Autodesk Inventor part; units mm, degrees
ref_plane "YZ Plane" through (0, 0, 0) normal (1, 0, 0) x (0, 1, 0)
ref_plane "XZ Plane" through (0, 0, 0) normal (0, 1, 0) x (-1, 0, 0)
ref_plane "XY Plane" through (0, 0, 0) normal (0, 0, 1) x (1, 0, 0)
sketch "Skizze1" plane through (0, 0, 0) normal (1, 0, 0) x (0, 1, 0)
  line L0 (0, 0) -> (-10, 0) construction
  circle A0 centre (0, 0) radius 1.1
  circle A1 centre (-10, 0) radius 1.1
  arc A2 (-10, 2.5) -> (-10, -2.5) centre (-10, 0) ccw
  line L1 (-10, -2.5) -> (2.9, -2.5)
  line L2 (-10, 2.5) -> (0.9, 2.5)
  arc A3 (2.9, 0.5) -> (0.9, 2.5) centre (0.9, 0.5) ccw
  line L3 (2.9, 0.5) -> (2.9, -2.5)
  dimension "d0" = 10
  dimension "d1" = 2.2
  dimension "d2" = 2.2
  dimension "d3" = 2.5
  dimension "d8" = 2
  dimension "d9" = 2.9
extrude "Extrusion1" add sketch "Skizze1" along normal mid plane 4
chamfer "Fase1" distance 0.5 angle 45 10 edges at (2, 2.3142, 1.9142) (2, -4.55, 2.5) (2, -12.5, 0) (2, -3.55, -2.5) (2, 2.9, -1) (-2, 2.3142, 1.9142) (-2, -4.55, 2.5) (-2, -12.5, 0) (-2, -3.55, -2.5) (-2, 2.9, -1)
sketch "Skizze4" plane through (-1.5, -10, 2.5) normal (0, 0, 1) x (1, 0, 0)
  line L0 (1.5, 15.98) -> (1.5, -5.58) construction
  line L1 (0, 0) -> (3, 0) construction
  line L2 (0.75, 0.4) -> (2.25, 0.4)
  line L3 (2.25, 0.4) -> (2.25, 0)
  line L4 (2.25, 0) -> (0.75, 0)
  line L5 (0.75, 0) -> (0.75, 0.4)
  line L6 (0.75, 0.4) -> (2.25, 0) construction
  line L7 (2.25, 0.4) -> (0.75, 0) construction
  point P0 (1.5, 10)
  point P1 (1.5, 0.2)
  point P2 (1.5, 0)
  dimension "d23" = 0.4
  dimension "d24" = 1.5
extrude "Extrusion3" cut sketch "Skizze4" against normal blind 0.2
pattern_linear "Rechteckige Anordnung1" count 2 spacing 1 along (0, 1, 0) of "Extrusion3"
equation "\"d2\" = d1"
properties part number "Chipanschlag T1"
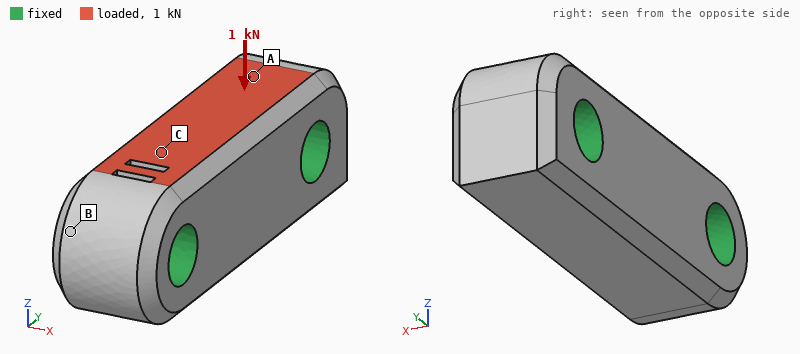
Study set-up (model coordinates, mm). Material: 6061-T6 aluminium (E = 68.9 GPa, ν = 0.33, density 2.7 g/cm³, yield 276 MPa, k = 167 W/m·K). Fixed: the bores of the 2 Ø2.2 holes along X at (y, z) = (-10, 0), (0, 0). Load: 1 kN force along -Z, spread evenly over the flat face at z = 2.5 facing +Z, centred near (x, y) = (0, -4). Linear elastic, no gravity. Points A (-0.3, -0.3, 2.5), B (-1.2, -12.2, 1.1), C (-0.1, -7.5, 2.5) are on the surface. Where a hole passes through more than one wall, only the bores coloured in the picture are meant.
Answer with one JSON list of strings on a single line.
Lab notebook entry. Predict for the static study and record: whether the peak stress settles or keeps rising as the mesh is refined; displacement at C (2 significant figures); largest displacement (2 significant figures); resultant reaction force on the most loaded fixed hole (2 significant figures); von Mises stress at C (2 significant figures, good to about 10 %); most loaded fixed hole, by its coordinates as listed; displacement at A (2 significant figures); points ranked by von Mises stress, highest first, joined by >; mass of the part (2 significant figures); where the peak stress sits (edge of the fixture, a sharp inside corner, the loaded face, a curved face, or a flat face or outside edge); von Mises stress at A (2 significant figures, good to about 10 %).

["keeps rising", "2.6 µm", "3.6 µm", "570 N", "18 MPa", "(0, 0)", "1.1 µm", "A > C > B", "0.69 g", "edge of the fixture", "37 MPa"]
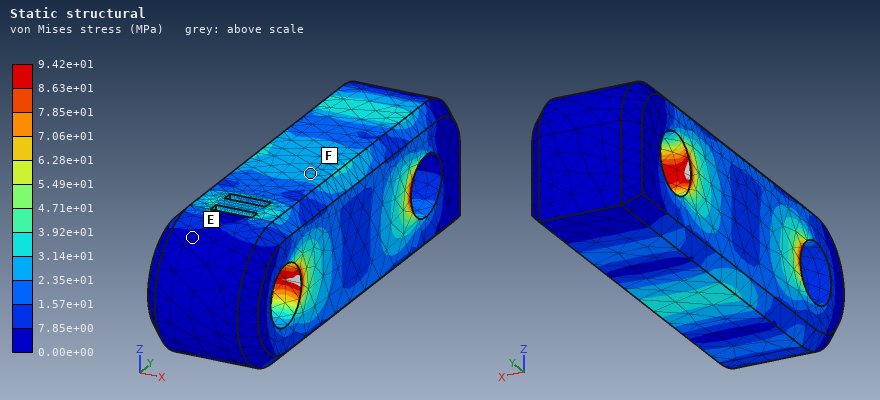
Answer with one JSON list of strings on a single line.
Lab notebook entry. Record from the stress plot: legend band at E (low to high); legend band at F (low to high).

["0.00e+00 to 7.85e+00 MPa", "2.35e+01 to 3.14e+01 MPa"]
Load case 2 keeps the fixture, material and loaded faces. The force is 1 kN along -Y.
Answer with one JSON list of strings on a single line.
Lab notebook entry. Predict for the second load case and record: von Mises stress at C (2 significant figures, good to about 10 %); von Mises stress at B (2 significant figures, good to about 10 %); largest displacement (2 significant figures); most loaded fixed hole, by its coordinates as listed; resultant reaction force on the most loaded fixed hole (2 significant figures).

["57 MPa", "8.0 MPa", "2.5 µm", "(0, 0)", "580 N"]
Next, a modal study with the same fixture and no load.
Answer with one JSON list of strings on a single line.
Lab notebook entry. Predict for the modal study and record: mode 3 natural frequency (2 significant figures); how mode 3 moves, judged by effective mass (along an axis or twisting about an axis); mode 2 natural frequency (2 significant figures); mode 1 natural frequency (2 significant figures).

["160 kHz", "twisting about Y", "140 kHz", "140 kHz"]
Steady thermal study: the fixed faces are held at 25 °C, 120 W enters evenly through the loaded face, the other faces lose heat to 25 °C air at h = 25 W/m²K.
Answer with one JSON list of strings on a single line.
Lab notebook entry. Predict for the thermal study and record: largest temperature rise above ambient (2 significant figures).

["69 K"]
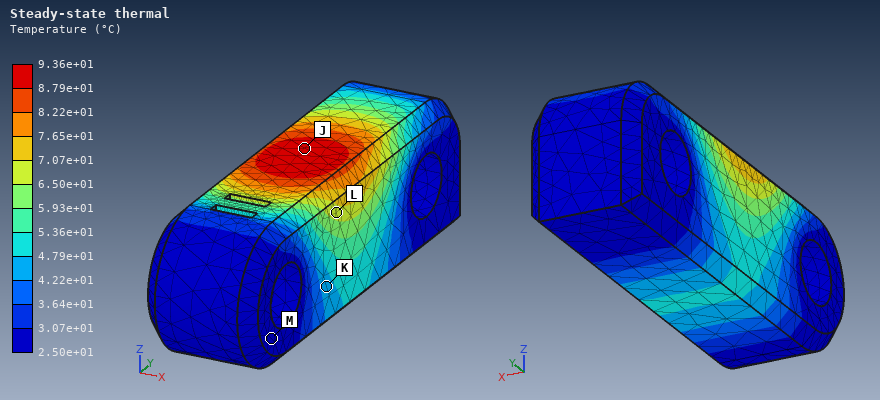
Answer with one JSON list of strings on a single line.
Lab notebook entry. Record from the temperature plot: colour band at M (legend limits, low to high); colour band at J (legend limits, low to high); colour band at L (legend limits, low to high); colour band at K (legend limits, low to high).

["2.50e+01 to 3.07e+01 °C", "8.79e+01 to 9.36e+01 °C", "6.50e+01 to 7.07e+01 °C", "4.22e+01 to 4.79e+01 °C"]
